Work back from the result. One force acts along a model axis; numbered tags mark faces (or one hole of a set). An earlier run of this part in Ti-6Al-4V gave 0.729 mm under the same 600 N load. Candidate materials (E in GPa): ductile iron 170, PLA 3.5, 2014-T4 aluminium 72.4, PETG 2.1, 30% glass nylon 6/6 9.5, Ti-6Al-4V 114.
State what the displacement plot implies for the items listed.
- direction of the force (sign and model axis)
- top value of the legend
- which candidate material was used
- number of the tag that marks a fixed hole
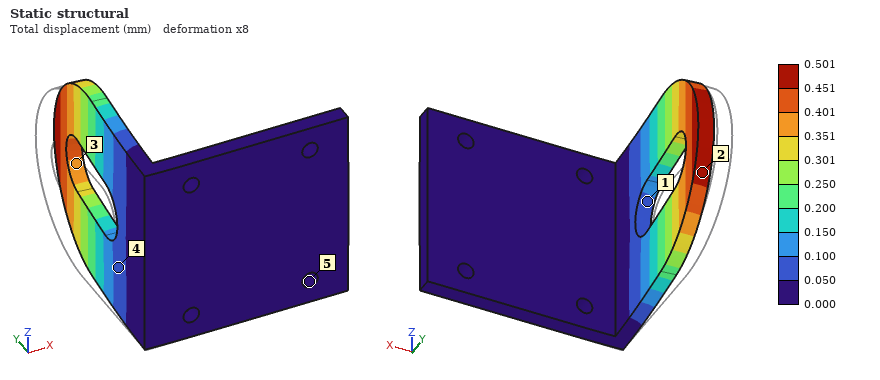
+X
0.501 mm
ductile iron
5
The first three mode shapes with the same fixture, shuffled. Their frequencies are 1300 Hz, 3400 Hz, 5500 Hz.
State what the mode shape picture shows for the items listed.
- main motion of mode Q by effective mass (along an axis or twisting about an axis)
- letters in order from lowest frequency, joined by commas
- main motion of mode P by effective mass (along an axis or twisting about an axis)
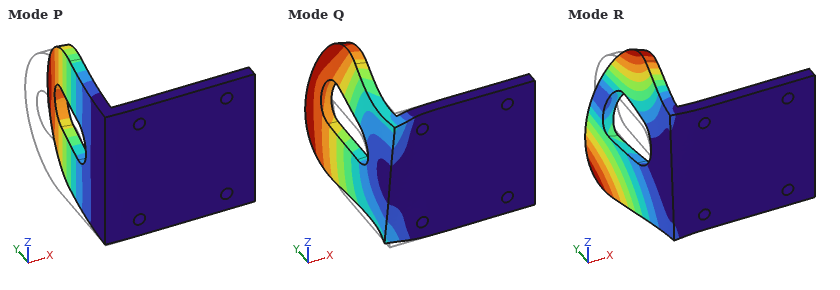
along Z
P, R, Q
along X
